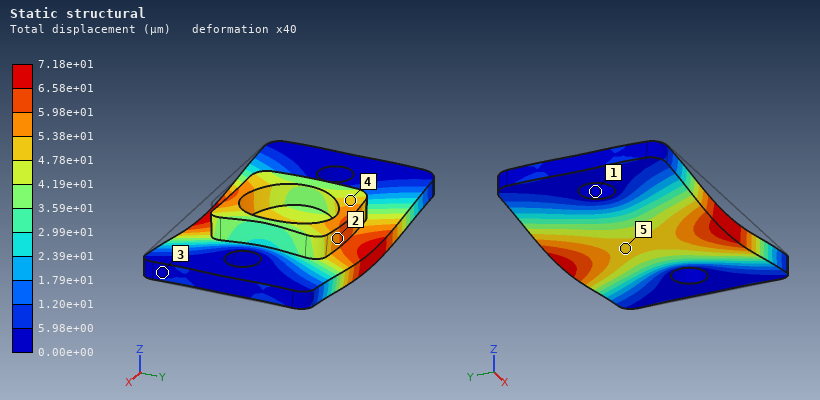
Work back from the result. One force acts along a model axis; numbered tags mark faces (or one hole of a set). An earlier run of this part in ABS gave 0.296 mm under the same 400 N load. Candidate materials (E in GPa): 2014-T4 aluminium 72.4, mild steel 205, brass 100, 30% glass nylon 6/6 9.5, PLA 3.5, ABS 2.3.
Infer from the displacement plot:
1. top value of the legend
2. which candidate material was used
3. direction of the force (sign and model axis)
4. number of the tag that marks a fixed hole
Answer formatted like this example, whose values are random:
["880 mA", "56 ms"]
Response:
["7.18e+01 µm", "30% glass nylon 6/6", "-Z", "1"]
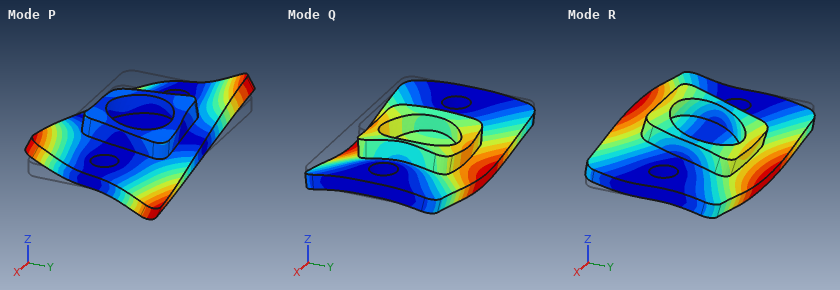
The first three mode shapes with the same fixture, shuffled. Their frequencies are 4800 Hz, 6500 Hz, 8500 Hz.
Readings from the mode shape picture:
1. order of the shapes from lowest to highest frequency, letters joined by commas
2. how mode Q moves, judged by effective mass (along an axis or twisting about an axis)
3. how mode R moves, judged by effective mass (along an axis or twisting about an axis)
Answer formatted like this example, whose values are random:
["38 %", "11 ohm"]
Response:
["R, Q, P", "along Z", "twisting about X"]
